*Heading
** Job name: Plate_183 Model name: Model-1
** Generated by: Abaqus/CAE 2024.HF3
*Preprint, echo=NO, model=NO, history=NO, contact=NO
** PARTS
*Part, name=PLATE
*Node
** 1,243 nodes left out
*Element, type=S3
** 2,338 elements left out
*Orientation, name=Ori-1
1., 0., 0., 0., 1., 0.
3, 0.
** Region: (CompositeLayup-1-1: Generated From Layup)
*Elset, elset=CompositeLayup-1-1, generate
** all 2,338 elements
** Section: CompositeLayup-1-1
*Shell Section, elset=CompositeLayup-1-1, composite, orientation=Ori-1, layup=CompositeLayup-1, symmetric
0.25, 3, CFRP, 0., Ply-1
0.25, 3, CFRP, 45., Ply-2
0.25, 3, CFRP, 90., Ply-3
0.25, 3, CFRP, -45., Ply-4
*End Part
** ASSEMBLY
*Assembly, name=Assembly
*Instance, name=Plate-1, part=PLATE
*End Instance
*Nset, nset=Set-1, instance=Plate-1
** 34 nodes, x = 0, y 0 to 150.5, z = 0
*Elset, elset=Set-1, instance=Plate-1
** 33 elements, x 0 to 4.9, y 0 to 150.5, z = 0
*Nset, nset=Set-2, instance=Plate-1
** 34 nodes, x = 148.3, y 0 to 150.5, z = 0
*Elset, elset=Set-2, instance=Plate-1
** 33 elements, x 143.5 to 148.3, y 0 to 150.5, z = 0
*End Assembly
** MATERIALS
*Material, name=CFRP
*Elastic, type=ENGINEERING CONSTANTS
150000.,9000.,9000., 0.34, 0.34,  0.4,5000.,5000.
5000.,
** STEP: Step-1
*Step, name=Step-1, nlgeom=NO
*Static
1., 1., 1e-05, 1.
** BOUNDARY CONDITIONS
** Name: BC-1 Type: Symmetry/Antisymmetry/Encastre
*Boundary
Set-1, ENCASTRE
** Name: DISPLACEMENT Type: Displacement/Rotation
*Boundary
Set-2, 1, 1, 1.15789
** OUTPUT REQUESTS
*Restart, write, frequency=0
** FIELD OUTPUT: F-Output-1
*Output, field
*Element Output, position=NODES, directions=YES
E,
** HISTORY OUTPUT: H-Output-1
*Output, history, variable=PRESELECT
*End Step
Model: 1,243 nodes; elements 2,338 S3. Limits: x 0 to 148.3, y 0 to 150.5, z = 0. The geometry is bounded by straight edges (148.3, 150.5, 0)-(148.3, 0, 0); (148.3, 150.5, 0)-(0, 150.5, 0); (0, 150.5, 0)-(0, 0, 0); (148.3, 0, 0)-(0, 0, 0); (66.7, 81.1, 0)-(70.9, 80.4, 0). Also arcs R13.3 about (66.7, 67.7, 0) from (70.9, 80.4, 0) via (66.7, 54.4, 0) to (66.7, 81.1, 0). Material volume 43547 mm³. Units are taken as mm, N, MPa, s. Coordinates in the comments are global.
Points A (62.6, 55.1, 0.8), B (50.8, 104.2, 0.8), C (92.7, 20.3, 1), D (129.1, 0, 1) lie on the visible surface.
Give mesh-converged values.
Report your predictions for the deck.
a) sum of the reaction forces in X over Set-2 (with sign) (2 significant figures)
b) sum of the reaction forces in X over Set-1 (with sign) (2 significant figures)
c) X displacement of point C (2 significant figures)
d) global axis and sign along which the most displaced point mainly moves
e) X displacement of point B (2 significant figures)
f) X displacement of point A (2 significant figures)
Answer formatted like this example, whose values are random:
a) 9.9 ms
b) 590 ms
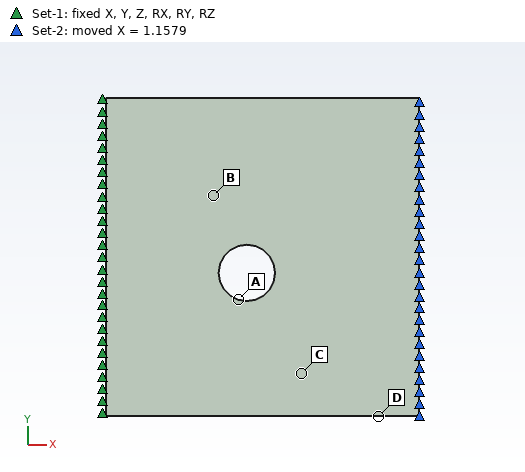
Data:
a) 1.3e+05 N
b) -1.3e+05 N
c) 0.73 mm
d) +X
e) 0.38 mm
f) 0.42 mm
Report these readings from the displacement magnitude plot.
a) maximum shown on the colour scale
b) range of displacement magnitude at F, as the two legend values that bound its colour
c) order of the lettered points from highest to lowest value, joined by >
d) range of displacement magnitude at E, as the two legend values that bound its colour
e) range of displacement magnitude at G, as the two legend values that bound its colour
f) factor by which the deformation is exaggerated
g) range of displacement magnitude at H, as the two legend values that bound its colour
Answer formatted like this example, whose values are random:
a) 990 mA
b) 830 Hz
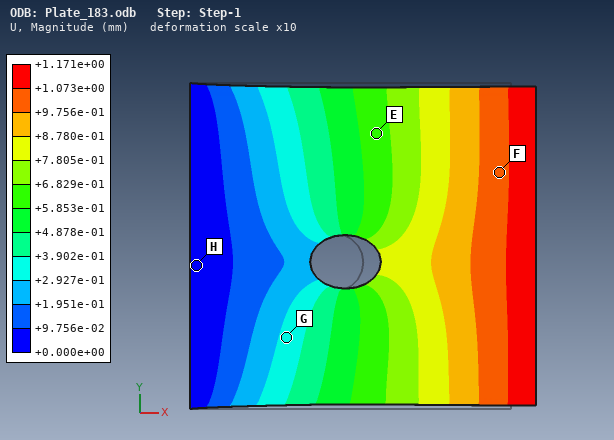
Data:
a) +1.171e+00 mm
b) +9.756e-01 to +1.073e+00 mm
c) F > E > G > H
d) +5.853e-01 to +6.829e-01 mm
e) +2.927e-01 to +3.902e-01 mm
f) 10
g) +0.000e+00 to +9.756e-02 mm
